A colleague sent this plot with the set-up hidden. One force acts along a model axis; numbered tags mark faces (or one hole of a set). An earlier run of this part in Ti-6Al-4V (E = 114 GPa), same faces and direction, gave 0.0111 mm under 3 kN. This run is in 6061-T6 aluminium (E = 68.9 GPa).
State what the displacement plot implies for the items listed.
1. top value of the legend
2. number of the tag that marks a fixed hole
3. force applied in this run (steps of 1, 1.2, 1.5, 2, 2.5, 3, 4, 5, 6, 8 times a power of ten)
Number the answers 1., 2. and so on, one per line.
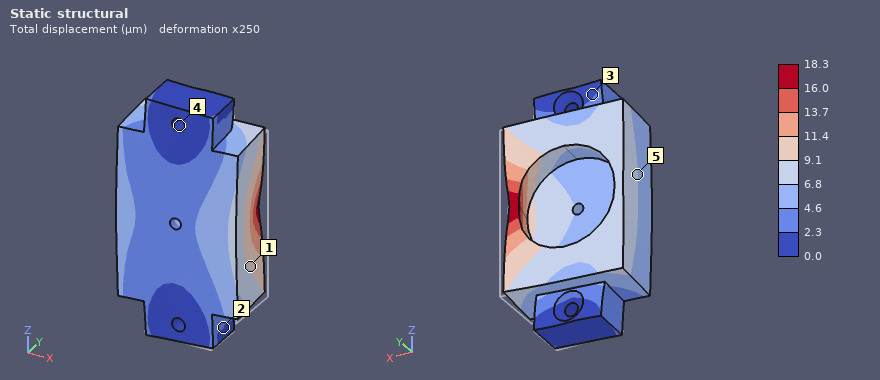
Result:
1. 18.3 µm
2. 4
3. 3 kN
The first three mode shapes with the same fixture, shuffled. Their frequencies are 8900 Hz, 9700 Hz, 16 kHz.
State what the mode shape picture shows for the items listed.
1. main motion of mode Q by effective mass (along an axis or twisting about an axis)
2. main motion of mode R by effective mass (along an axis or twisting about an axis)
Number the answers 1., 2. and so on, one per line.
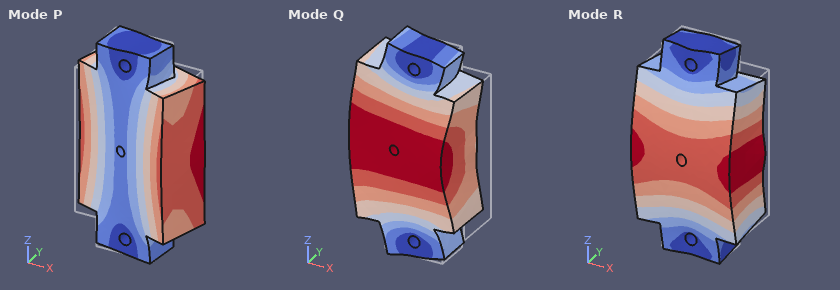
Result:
1. along X
2. along Y
